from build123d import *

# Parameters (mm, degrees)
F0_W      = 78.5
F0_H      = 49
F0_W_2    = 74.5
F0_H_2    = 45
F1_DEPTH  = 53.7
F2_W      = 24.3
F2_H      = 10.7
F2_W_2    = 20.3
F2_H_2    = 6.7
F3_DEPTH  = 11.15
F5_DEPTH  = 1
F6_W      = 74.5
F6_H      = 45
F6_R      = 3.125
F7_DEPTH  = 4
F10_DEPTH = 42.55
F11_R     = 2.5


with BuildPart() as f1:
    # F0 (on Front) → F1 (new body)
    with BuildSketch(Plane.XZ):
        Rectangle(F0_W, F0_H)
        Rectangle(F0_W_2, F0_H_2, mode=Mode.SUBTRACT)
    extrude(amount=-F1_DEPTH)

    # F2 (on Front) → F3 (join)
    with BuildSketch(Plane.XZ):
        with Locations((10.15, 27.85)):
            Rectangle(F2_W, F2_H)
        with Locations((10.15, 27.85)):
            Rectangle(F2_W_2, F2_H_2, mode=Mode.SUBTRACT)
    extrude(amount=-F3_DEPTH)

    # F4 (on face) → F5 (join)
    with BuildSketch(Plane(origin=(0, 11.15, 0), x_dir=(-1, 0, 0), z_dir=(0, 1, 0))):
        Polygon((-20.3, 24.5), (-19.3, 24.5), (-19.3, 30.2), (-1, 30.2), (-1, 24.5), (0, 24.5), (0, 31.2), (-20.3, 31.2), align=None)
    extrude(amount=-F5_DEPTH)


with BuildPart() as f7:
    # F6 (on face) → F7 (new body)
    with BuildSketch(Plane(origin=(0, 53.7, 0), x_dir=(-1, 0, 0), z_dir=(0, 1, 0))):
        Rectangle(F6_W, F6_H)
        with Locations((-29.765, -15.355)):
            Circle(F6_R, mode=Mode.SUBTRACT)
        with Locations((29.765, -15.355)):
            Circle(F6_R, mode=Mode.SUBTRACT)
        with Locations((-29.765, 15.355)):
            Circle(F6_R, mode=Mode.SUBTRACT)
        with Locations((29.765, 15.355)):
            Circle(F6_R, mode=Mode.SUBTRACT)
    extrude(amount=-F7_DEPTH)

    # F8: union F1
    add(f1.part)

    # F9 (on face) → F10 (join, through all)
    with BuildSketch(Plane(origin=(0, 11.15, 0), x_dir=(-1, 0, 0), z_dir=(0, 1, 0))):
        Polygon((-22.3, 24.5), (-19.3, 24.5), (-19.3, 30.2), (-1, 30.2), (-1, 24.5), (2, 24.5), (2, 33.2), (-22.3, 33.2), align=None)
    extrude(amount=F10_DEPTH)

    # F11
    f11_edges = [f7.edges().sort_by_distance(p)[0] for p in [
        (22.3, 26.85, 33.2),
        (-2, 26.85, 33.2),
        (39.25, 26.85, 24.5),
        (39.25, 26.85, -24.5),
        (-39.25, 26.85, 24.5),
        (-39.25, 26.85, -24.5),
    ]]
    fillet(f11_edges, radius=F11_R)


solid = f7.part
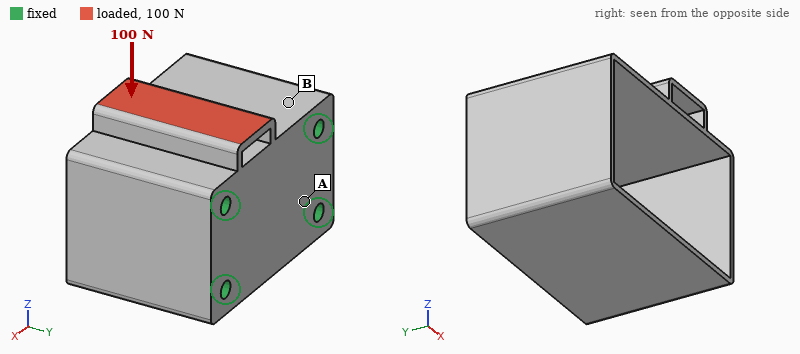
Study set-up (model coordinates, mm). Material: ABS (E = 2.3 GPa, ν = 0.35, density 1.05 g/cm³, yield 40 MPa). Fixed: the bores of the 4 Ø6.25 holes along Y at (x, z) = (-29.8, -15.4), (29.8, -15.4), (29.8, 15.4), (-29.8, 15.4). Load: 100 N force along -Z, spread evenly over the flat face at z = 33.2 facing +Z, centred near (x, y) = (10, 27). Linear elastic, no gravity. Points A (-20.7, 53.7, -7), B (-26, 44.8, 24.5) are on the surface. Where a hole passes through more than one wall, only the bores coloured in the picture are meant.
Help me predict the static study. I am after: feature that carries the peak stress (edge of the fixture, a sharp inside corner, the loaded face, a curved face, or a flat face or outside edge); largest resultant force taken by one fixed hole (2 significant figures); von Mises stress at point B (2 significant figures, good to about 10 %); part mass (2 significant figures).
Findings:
a flat face or outside edge
59 N
2.9 MPa
47 g
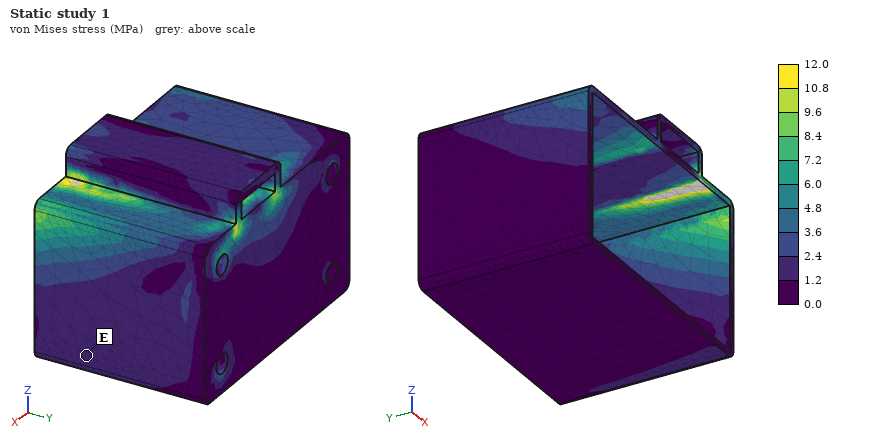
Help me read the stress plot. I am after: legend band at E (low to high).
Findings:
1.2 to 2.4 MPa
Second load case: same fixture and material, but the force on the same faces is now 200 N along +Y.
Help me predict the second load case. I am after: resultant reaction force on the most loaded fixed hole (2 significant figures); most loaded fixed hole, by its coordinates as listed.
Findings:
190 N
(29.8, 15.4)
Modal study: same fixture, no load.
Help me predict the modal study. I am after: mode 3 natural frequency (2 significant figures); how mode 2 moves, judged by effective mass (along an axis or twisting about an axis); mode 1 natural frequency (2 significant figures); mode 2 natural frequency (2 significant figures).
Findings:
960 Hz
along Z
490 Hz
560 Hz
